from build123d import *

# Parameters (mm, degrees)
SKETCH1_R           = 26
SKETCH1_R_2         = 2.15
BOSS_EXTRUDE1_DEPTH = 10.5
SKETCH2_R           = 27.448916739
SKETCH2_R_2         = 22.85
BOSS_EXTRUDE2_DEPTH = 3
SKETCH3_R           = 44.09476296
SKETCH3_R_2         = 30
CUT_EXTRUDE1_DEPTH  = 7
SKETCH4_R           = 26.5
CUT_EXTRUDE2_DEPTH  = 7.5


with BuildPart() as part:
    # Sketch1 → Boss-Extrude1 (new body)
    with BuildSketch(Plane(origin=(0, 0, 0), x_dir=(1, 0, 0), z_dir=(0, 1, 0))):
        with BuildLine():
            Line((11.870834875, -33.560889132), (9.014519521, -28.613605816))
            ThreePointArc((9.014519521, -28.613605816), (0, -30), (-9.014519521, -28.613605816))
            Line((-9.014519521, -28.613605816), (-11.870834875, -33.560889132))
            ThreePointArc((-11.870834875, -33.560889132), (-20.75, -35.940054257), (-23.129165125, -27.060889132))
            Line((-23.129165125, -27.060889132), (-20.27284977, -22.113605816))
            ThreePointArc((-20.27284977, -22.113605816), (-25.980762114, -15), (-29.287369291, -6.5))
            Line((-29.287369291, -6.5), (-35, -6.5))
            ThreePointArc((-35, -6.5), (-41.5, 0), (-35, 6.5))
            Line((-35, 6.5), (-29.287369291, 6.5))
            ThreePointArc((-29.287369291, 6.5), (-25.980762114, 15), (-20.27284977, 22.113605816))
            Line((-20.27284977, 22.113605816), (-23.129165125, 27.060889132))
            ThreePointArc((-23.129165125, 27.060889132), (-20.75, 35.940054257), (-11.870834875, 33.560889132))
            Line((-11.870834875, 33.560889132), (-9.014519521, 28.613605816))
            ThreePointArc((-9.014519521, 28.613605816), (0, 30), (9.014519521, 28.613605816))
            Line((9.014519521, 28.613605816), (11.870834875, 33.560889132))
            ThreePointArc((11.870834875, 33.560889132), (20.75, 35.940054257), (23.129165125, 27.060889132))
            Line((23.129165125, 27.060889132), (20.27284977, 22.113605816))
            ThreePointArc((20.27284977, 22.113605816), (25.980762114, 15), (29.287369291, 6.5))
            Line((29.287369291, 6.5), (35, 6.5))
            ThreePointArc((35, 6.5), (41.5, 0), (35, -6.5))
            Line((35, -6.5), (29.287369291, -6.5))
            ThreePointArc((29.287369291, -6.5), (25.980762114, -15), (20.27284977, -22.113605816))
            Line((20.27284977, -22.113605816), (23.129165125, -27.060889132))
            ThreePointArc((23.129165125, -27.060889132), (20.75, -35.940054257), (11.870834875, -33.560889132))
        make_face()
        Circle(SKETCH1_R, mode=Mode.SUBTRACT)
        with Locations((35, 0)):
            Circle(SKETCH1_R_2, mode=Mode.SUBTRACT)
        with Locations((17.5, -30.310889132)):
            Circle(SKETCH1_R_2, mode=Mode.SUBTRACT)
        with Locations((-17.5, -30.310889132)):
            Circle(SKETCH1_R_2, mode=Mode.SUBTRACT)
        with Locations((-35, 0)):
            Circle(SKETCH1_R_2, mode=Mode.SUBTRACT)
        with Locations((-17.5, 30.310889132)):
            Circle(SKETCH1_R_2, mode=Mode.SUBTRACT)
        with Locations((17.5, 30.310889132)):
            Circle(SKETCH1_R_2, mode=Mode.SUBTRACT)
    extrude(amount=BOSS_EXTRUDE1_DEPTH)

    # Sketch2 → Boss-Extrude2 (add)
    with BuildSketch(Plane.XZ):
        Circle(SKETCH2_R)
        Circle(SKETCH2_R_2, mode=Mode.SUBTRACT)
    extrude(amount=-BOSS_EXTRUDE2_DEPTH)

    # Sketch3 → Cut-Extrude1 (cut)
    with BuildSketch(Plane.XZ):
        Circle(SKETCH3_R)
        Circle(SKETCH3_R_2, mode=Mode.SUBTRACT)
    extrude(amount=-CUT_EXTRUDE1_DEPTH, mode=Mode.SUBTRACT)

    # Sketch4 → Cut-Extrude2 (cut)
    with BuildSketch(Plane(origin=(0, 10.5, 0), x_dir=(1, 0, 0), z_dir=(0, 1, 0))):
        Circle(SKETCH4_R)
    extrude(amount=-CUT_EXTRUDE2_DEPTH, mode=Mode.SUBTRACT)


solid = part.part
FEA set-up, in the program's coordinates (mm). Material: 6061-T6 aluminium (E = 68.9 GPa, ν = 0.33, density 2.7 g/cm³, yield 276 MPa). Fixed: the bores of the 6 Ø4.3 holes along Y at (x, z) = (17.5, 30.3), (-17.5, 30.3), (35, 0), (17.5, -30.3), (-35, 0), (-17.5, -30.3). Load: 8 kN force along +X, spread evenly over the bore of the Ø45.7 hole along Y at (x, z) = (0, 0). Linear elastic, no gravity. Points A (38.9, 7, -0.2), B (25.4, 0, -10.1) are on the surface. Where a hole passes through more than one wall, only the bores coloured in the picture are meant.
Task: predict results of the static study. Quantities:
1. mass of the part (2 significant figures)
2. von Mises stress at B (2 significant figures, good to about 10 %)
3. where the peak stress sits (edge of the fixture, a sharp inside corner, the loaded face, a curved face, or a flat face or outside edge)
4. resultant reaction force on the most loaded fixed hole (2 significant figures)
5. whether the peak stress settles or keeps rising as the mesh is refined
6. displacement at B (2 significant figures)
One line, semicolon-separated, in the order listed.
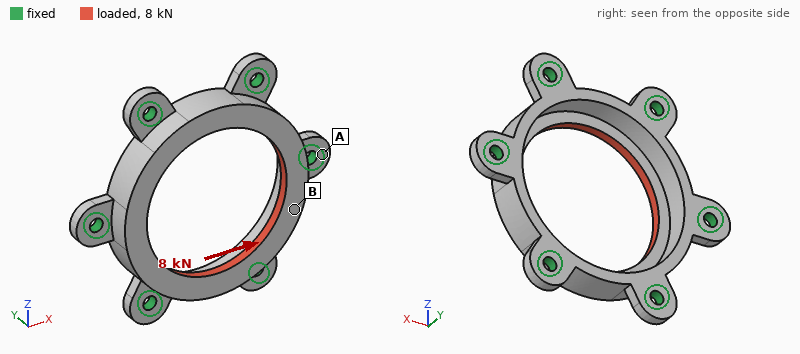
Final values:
29 g; 57 MPa; edge of the fixture; 1.5 kN; keeps rising; 41 µm
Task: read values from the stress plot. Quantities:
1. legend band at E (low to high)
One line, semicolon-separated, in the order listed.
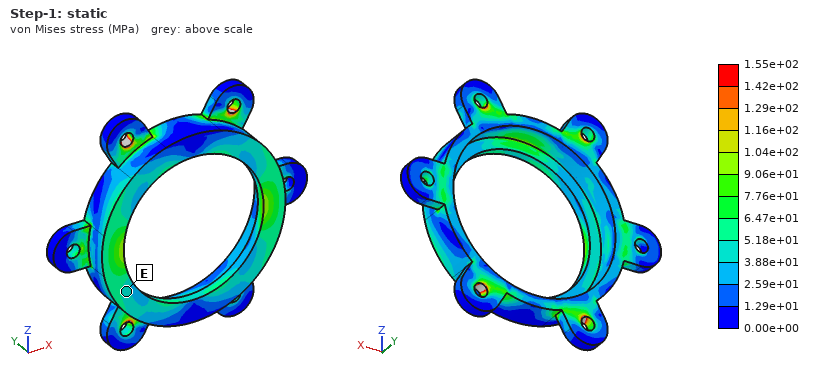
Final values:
3.88e+01 to 5.18e+01 MPa
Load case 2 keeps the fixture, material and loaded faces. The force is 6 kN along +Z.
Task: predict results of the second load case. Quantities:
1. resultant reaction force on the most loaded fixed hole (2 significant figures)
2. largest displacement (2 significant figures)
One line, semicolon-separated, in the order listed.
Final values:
1.2 kN; 40 µm
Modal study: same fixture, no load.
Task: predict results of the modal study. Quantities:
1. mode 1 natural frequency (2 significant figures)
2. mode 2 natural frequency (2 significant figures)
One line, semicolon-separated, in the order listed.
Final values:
18 kHz; 18 kHz
